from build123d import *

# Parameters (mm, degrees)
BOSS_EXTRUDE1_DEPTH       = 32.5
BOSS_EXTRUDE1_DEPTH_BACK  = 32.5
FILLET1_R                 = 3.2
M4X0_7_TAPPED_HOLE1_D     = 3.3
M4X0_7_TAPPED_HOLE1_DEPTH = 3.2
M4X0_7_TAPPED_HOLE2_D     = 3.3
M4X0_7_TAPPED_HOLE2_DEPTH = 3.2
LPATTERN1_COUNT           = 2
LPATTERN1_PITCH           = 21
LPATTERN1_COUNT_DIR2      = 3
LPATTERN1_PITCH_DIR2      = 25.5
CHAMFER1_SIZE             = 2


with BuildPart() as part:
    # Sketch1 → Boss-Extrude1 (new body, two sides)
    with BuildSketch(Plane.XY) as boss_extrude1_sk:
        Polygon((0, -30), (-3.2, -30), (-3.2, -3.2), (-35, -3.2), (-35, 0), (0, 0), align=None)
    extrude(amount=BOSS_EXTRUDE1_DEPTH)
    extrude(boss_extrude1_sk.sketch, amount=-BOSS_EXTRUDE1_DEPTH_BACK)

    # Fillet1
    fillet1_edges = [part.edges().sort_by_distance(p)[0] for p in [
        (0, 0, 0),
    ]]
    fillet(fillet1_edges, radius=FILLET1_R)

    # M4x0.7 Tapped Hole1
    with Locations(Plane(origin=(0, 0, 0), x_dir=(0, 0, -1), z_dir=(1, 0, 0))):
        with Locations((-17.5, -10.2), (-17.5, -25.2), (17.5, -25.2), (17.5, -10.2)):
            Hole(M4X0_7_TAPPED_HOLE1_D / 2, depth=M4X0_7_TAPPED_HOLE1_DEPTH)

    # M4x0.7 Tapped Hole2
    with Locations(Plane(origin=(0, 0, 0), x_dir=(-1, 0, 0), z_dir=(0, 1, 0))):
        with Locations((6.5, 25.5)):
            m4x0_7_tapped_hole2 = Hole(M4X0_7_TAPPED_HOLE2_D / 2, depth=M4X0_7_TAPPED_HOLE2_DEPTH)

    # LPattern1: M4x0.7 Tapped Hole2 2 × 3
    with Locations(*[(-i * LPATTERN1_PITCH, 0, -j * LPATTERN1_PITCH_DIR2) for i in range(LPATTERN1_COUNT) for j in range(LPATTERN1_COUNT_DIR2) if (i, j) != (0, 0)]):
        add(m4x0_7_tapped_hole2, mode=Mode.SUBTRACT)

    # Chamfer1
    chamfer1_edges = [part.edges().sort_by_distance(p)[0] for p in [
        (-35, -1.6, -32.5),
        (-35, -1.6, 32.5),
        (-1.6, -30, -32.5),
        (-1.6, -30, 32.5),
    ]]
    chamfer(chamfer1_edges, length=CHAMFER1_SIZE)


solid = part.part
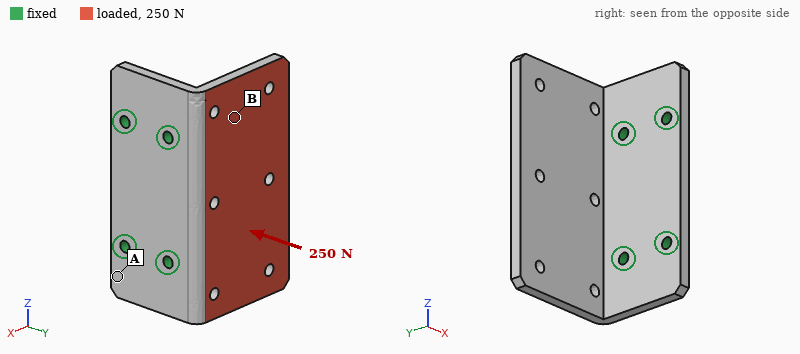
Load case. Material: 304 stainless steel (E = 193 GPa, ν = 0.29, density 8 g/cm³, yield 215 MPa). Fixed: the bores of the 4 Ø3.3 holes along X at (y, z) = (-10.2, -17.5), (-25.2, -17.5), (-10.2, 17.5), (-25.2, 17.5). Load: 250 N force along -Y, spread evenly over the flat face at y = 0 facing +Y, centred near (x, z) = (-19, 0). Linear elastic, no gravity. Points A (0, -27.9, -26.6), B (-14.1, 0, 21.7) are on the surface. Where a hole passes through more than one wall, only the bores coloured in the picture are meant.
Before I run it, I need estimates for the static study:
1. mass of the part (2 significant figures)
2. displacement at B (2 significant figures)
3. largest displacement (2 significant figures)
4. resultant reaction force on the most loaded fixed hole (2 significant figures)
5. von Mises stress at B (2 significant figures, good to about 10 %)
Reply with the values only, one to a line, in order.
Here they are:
99 g
24 µm
74 µm
110 N
14 MPa
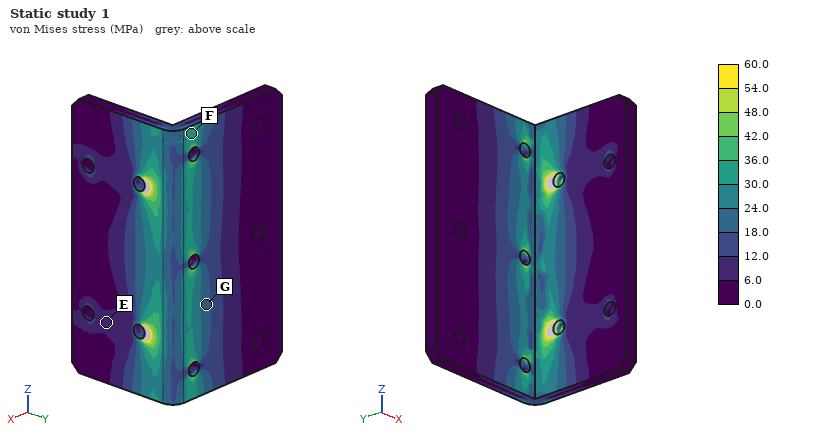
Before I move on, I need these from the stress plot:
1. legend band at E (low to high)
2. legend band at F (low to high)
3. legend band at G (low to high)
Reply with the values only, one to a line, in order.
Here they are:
6.0 to 12.0 MPa
30.0 to 36.0 MPa
18.0 to 24.0 MPa
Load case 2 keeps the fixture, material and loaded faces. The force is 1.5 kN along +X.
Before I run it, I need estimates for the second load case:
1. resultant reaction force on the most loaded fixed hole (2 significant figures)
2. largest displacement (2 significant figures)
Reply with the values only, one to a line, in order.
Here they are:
940 N
0.12 mm
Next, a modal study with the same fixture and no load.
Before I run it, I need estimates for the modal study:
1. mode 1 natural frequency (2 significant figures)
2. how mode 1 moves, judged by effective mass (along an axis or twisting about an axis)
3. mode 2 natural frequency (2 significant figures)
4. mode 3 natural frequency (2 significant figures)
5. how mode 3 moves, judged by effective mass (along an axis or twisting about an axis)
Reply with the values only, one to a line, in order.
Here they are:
1600 Hz
along Y
2900 Hz
5600 Hz
along Z
